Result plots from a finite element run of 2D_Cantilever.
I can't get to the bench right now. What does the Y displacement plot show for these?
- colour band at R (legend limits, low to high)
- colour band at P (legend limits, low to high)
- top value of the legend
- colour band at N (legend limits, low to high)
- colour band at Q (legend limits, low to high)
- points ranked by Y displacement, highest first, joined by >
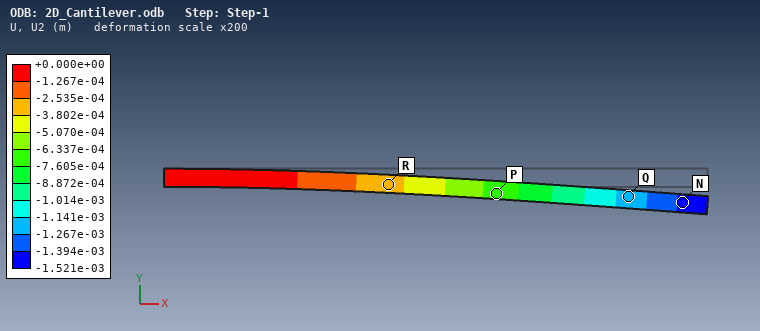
-3.802e-04 to -2.535e-04 m
-7.605e-04 to -6.337e-04 m
+0.000e+00 m
-1.521e-03 to -1.394e-03 m
-1.267e-03 to -1.141e-03 m
R > P > Q > N
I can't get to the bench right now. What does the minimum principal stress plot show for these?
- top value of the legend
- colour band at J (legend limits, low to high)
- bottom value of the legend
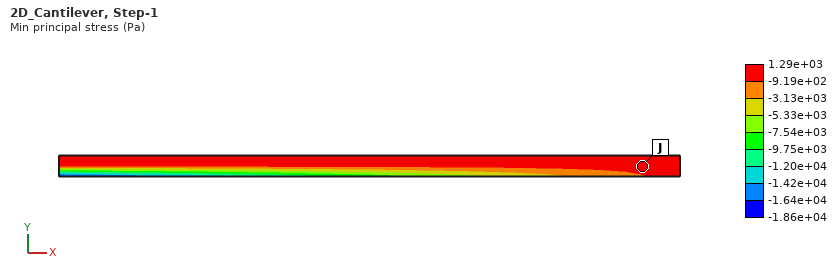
1.29e+03 Pa
-9.19e+02 to 1.29e+03 Pa
-1.86e+04 Pa
